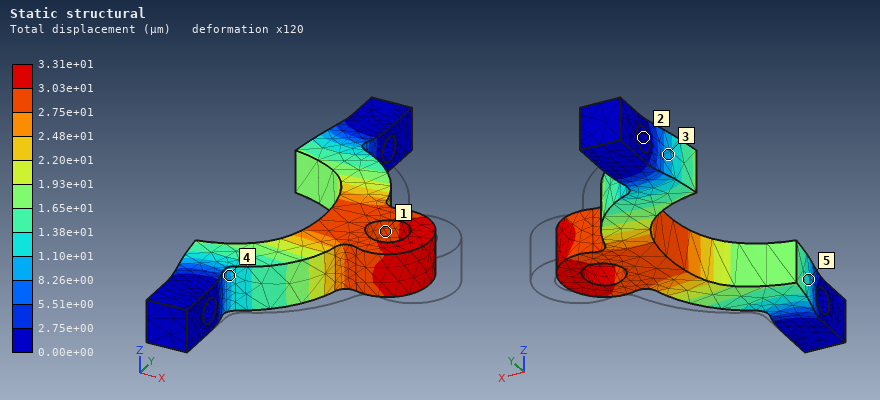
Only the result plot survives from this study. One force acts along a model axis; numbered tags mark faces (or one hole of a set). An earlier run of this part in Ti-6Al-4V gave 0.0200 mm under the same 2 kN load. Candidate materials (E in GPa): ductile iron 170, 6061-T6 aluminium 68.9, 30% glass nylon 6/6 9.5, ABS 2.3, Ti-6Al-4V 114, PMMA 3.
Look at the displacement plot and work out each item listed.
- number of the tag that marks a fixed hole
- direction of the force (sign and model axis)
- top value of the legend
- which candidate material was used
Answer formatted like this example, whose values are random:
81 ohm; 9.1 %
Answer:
2; -X; 3.31e+01 µm; 6061-T6 aluminium
